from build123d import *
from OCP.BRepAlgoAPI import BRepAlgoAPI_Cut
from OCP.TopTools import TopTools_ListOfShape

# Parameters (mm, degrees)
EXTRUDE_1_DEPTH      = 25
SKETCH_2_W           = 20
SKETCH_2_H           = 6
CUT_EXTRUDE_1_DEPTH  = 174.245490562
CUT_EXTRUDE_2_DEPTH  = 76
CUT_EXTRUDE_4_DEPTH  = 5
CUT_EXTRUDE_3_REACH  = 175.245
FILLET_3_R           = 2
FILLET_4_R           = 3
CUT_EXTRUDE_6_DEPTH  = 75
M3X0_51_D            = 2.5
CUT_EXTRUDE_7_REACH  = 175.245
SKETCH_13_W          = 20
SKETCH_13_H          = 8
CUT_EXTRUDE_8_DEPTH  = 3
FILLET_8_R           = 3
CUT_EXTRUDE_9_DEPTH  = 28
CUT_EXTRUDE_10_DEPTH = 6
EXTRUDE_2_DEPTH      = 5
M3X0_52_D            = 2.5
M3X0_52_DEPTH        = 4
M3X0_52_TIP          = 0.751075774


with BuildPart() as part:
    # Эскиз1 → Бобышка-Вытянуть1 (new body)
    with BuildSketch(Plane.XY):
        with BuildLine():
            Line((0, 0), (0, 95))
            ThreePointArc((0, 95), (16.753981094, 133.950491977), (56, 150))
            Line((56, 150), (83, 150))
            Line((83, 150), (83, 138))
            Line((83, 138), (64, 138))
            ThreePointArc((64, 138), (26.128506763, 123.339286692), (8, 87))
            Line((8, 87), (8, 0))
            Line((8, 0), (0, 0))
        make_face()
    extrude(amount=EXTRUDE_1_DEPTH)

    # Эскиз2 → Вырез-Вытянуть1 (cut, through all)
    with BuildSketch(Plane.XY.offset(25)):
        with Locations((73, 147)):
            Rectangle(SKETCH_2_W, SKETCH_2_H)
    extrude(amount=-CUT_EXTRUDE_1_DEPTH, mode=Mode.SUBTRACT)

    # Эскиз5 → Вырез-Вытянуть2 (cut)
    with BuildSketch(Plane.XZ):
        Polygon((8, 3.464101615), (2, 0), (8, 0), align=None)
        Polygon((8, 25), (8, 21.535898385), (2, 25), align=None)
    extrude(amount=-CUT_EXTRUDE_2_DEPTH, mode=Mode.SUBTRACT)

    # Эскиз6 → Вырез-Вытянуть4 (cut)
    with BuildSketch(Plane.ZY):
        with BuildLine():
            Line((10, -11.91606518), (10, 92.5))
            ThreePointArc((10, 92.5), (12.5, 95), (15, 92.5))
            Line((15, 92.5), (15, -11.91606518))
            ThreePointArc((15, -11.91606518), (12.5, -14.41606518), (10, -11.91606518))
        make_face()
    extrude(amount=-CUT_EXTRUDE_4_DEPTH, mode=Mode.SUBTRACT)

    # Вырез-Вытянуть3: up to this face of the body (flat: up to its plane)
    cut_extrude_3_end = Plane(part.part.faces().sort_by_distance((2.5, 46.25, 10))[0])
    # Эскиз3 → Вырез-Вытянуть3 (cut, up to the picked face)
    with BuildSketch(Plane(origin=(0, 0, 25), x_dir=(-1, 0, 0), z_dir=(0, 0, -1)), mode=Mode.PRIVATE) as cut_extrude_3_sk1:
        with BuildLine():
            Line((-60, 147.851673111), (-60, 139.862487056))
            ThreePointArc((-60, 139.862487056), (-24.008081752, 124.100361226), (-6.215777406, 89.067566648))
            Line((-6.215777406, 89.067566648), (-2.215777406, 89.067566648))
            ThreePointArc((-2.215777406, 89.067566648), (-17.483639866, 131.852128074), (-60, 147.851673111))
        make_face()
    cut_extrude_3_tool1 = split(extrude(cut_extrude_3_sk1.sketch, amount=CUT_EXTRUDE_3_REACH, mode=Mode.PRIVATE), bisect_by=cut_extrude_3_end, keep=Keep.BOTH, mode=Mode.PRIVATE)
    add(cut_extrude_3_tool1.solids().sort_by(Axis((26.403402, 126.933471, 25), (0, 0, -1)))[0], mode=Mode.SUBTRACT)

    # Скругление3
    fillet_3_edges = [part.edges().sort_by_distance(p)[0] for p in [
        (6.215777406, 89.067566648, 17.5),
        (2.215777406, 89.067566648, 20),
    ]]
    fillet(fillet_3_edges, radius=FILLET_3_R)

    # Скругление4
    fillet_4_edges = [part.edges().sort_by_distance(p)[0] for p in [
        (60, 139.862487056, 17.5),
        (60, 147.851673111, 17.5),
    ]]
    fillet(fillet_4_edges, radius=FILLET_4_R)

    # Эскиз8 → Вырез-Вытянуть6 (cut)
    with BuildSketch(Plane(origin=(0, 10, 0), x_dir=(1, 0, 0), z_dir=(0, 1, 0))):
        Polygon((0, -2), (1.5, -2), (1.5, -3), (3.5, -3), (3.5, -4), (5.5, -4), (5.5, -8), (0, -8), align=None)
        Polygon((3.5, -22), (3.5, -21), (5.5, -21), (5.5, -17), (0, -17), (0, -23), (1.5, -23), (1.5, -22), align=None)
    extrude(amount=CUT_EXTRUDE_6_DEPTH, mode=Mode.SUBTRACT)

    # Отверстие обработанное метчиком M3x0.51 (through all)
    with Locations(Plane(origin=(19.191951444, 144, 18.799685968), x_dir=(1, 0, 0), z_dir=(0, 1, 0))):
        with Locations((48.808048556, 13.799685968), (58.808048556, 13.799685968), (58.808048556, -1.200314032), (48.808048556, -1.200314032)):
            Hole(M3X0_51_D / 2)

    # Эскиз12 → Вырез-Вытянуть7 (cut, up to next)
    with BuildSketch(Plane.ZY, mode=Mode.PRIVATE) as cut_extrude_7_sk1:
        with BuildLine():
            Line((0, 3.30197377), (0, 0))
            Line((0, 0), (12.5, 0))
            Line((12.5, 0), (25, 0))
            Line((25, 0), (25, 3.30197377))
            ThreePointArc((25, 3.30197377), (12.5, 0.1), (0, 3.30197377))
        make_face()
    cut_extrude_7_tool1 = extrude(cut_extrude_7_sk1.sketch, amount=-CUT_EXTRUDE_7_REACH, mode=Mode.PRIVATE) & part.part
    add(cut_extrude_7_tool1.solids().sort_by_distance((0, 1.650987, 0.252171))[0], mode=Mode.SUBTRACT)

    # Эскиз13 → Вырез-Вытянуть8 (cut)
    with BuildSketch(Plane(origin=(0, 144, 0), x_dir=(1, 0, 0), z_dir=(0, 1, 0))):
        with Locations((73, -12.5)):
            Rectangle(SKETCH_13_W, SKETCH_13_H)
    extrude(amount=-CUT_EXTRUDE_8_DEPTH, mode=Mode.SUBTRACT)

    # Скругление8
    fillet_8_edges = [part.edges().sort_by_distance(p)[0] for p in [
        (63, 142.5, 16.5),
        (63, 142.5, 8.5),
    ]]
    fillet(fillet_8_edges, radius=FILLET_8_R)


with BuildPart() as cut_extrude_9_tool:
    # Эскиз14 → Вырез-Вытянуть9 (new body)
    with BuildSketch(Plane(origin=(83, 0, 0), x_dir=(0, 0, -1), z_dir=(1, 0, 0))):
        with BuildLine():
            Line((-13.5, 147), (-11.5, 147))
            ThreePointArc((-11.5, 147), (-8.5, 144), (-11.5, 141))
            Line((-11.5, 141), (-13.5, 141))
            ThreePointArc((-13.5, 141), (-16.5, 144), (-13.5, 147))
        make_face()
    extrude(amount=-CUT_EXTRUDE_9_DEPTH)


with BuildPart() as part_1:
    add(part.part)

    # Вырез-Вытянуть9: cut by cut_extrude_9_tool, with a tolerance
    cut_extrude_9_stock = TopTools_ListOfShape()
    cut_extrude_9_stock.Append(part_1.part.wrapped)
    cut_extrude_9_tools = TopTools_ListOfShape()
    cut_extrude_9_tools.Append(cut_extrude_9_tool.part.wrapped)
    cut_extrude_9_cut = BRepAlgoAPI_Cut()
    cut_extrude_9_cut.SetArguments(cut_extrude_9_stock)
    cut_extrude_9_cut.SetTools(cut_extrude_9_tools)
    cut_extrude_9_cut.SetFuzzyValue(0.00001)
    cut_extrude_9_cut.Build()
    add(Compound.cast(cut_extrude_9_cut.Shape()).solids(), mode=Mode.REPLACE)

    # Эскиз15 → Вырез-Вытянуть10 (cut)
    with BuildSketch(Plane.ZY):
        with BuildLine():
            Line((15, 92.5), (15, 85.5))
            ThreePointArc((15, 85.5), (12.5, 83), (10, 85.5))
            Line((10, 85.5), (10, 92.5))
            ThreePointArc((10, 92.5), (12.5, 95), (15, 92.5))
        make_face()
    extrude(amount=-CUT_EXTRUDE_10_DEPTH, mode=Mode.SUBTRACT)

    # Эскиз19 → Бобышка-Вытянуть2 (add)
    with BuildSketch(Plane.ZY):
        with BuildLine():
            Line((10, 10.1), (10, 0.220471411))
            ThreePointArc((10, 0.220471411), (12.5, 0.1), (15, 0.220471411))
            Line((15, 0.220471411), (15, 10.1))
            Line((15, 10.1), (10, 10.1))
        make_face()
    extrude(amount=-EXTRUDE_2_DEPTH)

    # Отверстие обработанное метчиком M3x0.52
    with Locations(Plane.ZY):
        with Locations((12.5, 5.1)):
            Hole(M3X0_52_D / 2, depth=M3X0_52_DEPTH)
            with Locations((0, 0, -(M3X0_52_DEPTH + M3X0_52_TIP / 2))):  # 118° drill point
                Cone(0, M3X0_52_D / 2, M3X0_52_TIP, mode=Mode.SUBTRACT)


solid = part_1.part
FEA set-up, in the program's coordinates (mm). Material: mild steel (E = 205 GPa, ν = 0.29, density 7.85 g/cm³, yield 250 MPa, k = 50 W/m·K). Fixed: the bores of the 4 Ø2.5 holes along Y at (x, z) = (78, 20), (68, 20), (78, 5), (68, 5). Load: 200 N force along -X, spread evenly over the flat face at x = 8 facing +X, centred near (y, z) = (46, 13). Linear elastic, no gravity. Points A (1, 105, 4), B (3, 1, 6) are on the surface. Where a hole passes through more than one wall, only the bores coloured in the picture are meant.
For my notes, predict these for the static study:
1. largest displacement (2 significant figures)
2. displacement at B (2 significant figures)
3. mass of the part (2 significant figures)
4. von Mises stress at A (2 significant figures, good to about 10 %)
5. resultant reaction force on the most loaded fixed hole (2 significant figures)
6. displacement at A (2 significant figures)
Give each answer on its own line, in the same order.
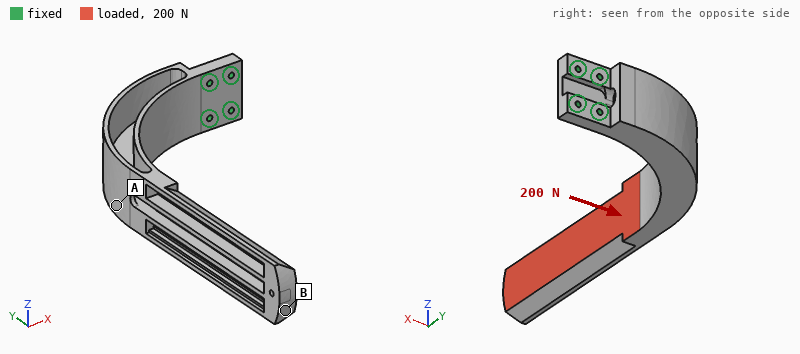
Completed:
0.88 mm
0.86 mm
230 g
31 MPa
340 N
0.26 mm
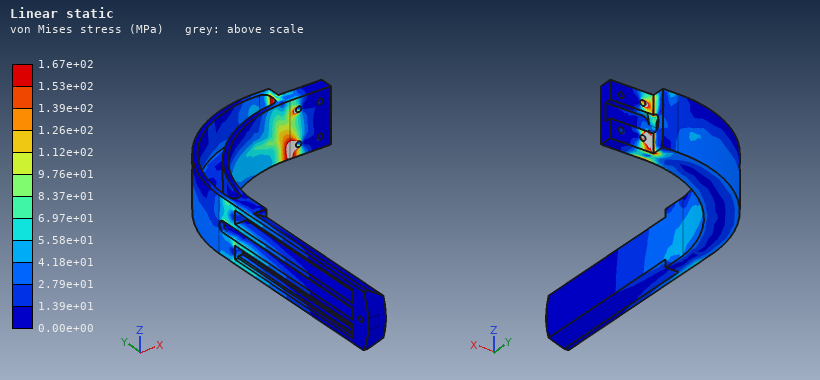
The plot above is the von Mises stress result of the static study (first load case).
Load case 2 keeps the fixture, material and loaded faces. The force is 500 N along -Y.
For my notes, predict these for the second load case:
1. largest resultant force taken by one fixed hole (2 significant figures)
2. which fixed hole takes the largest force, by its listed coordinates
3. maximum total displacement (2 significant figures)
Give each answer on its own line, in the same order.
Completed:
760 N
(68, 5)
0.75 mm
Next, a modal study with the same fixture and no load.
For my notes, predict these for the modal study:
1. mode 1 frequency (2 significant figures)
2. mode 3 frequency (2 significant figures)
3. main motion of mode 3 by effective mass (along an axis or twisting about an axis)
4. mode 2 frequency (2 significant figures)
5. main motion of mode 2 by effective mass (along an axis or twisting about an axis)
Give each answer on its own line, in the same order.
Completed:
280 Hz
910 Hz
along Y
390 Hz
along Z
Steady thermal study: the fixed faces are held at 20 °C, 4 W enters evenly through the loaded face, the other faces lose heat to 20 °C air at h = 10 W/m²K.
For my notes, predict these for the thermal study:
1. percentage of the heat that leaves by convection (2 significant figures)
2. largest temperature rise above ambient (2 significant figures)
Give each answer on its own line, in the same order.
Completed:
67 %
34 K
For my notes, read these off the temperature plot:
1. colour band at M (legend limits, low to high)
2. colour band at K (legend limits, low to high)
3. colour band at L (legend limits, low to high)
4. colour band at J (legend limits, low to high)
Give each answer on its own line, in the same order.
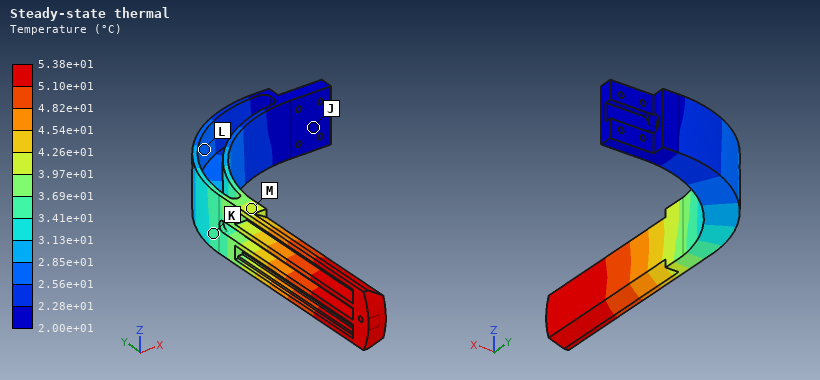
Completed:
3.97e+01 to 4.26e+01 °C
3.41e+01 to 3.69e+01 °C
2.56e+01 to 2.85e+01 °C
2.00e+01 to 2.28e+01 °C
